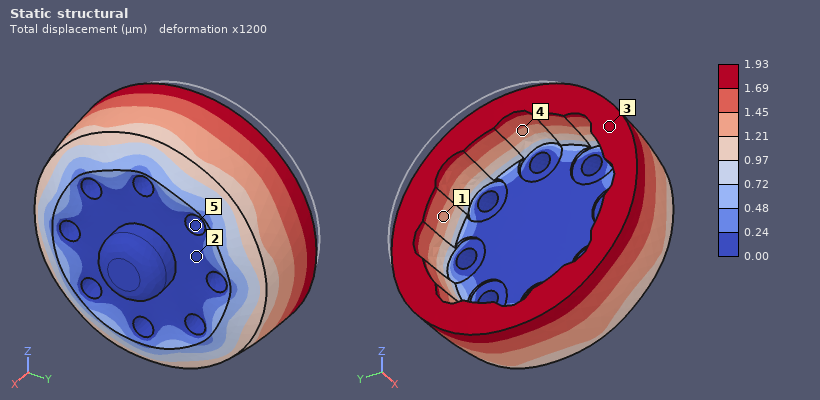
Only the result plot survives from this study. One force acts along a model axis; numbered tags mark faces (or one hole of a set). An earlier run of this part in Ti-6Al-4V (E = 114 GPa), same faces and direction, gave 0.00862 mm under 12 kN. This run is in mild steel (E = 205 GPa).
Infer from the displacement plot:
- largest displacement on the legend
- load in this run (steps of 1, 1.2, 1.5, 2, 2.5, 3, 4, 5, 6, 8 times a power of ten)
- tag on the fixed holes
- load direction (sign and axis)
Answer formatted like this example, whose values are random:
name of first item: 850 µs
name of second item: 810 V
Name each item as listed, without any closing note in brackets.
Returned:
largest displacement on the legend: 1.93 µm
load in this run: 5 kN
tag on the fixed holes: 5
load direction: +X
